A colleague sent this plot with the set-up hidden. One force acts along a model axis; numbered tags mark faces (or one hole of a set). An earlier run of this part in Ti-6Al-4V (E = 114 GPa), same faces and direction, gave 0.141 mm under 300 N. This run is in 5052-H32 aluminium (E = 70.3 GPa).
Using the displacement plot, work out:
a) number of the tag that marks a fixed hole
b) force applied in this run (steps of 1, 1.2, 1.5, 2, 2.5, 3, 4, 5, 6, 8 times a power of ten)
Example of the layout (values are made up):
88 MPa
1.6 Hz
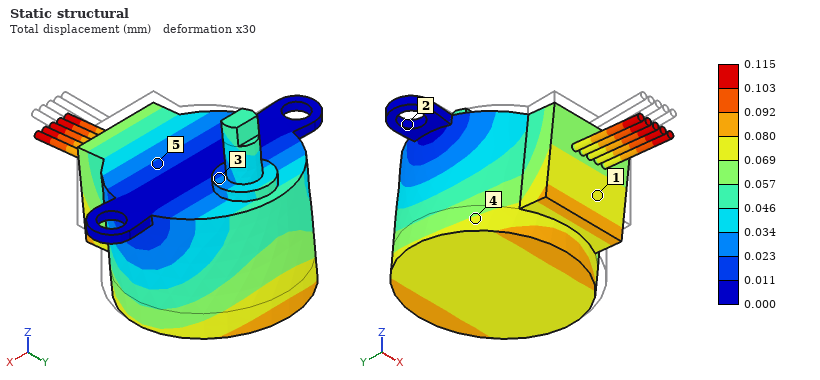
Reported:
2
150 N
